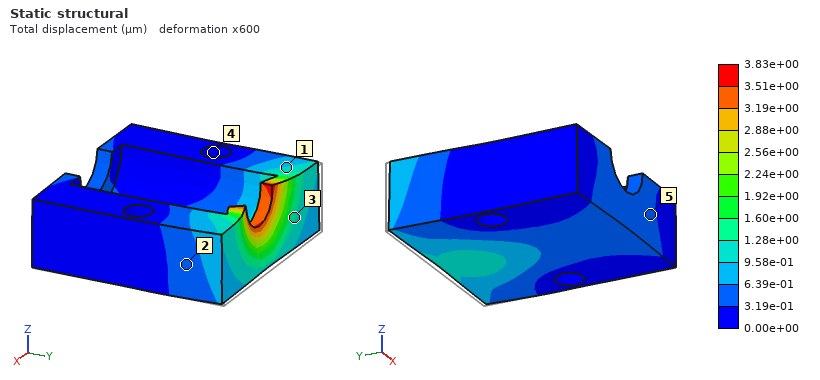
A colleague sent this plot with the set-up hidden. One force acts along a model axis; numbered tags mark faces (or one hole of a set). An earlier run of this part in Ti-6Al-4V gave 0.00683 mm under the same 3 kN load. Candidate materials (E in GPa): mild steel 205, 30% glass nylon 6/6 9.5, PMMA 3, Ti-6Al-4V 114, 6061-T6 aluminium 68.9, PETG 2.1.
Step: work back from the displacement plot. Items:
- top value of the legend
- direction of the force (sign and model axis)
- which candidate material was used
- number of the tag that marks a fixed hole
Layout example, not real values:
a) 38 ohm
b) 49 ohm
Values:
a) 3.83e+00 µm
b) -Y
c) mild steel
d) 4
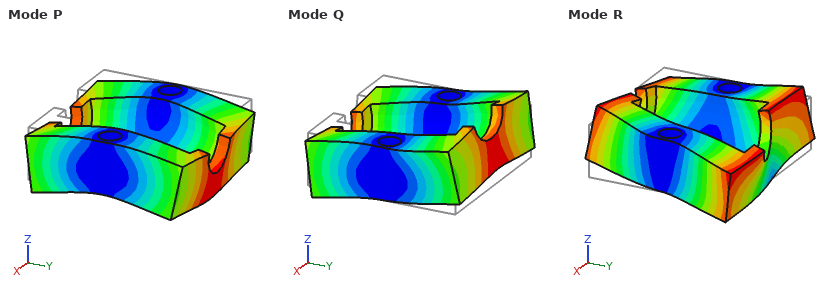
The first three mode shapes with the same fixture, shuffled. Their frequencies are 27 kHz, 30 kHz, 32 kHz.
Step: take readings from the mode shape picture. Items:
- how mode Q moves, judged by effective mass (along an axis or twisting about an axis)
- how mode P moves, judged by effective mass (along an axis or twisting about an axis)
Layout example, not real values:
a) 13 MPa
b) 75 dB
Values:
a) twisting about X
b) along Z
